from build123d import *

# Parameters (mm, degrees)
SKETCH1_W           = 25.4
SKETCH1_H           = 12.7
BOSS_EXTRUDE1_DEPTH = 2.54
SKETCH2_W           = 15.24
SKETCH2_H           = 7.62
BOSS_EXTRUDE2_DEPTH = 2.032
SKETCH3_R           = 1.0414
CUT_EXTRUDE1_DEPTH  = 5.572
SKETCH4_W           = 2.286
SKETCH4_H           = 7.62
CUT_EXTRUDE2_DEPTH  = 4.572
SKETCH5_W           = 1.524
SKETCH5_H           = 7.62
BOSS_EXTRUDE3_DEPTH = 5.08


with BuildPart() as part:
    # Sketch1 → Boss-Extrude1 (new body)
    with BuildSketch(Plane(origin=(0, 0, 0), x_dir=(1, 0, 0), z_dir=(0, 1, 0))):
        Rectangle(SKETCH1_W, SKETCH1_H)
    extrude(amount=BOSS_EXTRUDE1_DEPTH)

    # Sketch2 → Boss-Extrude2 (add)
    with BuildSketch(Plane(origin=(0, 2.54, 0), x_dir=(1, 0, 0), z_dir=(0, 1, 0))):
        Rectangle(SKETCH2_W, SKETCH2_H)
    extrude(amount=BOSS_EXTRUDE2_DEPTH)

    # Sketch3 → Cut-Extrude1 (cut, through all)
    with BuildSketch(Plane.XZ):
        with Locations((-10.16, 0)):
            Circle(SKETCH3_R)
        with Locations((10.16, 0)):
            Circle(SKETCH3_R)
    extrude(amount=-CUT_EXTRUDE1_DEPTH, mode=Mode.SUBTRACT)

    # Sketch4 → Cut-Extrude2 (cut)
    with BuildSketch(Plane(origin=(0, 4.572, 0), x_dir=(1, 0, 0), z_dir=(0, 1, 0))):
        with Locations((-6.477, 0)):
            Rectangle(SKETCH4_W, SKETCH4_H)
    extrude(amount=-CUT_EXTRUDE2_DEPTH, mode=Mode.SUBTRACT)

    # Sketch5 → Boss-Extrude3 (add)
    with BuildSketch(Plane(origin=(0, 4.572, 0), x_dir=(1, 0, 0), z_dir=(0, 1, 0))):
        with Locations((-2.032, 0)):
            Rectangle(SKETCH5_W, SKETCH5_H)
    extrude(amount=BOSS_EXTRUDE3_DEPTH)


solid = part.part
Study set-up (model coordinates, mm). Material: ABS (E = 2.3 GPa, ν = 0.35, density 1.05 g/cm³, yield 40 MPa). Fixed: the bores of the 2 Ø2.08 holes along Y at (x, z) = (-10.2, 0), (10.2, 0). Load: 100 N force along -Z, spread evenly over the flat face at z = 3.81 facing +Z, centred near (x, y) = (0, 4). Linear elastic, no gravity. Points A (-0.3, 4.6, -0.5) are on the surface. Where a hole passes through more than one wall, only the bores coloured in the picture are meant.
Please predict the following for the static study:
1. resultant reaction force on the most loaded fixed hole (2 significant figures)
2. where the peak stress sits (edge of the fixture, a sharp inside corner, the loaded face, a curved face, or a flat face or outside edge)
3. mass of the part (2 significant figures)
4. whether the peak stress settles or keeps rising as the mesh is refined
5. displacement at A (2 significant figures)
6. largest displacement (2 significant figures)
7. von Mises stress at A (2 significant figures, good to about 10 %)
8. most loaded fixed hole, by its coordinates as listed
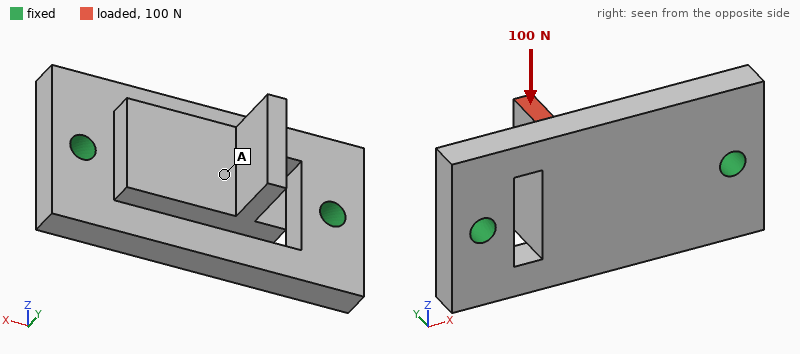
58 N
edge of the fixture
1.1 g
keeps rising
0.097 mm
0.22 mm
2.3 MPa
(10.2, 0)
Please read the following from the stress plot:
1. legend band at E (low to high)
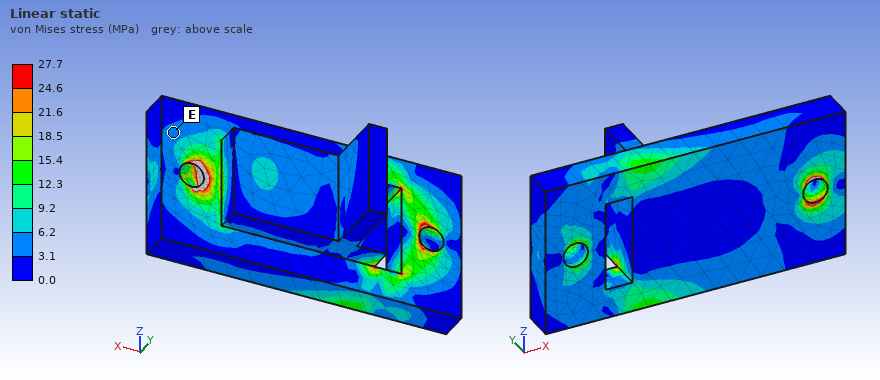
3.1 to 6.2 MPa
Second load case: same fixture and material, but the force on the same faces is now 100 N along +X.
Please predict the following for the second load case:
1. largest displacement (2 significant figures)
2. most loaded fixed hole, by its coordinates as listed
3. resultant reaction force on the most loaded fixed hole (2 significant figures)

0.27 mm
(10.2, 0)
86 N
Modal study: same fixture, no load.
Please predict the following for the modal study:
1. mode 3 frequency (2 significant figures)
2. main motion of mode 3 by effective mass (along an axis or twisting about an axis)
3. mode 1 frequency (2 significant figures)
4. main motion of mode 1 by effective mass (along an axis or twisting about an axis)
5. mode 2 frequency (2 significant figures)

9700 Hz
along Z
5500 Hz
along Y
6000 Hz
